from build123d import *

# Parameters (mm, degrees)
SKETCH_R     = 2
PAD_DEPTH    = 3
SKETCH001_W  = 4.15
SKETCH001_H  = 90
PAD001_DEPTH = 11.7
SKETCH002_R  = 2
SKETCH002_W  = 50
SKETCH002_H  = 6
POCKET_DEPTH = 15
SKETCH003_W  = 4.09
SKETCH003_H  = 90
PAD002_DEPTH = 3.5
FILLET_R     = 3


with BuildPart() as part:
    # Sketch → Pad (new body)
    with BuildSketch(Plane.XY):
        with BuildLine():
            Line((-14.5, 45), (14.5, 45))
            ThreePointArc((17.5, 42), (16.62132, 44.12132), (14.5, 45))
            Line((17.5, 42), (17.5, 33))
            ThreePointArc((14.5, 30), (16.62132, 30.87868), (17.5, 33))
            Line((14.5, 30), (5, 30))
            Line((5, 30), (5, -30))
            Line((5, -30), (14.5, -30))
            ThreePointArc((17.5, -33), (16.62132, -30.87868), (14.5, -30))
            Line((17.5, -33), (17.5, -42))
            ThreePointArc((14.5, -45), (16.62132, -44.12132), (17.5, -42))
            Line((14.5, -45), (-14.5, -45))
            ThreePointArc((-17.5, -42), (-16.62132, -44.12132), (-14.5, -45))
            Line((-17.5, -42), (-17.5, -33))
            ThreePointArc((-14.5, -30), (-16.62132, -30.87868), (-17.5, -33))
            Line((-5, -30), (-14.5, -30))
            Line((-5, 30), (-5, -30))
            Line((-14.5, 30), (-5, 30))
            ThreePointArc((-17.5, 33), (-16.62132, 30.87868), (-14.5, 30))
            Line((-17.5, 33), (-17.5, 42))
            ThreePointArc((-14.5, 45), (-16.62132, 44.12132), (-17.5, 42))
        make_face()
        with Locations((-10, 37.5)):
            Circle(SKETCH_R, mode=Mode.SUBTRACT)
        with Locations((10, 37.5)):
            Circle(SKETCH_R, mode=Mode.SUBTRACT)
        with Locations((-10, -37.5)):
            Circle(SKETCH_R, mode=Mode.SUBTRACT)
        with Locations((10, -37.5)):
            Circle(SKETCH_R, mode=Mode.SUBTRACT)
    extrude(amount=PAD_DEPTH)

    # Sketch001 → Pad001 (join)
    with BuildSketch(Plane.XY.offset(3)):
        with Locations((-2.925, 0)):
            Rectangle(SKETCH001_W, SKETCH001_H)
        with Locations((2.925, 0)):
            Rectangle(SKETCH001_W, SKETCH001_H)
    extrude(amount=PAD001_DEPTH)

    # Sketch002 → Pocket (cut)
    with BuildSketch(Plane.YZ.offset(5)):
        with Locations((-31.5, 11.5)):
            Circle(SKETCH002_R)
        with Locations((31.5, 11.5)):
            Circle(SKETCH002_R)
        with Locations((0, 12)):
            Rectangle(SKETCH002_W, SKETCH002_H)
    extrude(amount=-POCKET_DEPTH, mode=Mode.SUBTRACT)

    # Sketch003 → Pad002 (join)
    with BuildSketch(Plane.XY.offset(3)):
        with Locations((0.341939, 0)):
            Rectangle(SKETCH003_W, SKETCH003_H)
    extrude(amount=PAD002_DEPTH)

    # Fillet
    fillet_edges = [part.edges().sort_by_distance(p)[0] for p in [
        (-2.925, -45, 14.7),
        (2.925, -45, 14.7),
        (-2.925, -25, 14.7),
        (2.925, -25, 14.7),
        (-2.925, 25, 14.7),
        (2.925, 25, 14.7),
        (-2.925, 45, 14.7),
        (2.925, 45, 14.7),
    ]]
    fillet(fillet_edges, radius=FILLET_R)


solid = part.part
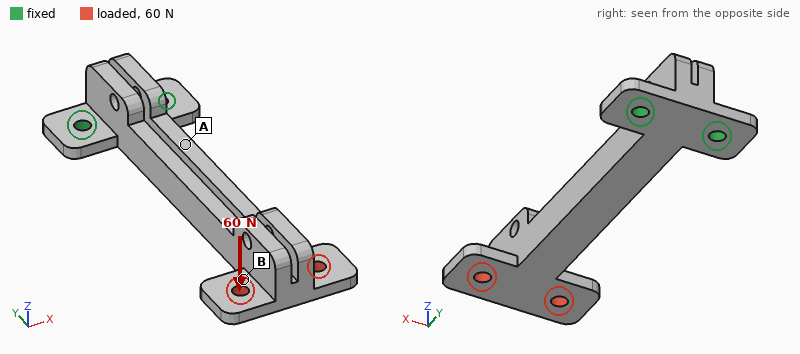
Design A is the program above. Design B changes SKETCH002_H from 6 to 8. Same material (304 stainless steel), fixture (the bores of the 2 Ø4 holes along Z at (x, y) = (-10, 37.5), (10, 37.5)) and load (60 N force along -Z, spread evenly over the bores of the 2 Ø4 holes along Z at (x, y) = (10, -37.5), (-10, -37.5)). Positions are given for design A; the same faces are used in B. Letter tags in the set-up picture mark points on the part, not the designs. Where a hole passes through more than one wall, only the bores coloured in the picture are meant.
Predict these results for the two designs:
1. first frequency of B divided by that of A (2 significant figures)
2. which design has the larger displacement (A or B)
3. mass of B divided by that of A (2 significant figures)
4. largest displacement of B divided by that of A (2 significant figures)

0.94
B
0.96
1.2
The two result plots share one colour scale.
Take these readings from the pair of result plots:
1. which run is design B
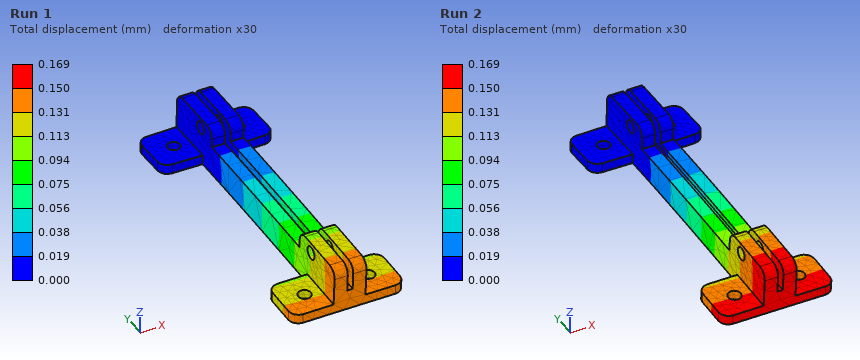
Run 2
